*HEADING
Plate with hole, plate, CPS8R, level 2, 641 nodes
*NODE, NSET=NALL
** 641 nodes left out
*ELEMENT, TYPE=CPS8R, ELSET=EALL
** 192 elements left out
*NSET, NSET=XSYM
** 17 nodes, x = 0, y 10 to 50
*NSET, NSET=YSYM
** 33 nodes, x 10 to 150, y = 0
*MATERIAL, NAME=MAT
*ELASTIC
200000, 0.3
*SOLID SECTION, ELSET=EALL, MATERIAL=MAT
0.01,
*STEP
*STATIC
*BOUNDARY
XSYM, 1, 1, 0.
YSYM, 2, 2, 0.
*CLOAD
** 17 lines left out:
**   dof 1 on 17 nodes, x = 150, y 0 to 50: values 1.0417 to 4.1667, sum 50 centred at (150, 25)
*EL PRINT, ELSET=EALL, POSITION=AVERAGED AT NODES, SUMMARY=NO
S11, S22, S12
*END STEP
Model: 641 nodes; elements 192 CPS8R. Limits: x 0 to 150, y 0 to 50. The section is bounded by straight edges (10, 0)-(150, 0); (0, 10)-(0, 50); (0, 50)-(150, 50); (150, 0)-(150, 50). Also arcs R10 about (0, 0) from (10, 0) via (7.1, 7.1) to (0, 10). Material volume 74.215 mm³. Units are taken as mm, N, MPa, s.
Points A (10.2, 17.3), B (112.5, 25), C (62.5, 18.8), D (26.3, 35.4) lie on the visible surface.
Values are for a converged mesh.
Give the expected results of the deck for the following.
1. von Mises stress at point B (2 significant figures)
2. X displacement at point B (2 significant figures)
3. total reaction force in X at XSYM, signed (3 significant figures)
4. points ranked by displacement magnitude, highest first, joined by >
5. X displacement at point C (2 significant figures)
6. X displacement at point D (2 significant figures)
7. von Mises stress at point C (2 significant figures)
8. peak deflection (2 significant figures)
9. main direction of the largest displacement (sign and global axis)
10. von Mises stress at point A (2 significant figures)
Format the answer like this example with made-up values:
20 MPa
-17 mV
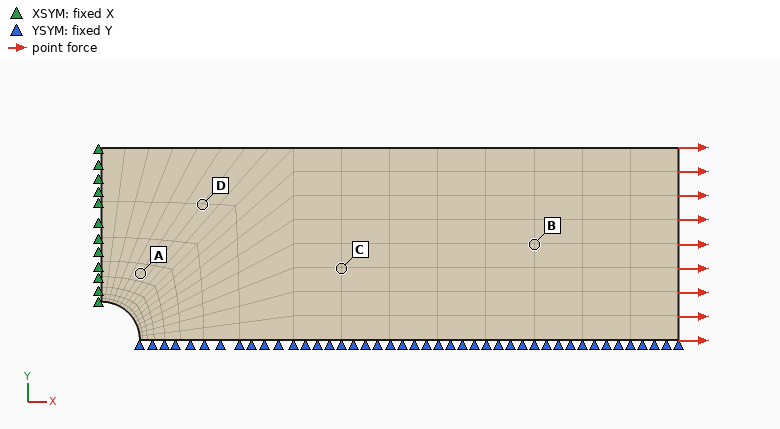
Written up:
100 MPa
0.059 mm
-50.0 N
B > C > D > A
0.034 mm
0.014 mm
97 MPa
0.079 mm
+X
130 MPa
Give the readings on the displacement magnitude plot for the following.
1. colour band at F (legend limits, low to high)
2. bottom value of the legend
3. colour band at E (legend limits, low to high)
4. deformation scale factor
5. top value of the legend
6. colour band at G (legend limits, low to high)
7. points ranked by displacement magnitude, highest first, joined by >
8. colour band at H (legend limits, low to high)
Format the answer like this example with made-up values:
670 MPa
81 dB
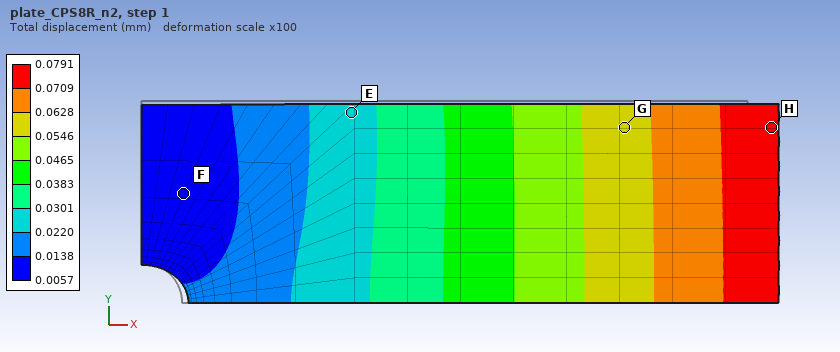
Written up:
0.0057 to 0.0138 mm
0.0057 mm
0.0220 to 0.0301 mm
100
0.0791 mm
0.0546 to 0.0628 mm
H > G > E > F
0.0709 to 0.0791 mm
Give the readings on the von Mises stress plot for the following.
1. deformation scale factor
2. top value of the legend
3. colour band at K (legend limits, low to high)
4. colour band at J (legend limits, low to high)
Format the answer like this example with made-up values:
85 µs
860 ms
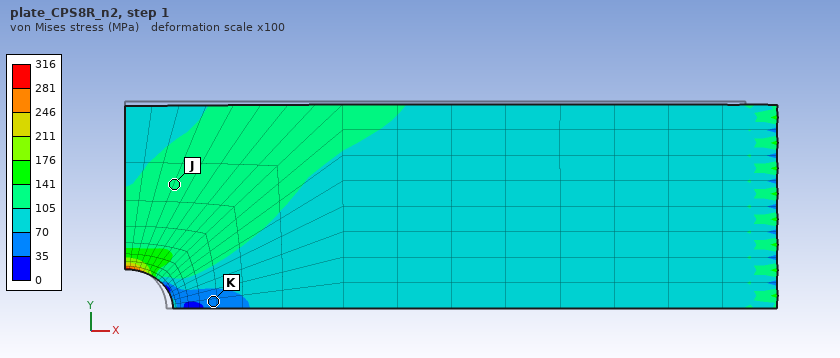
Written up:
100
316 MPa
35 to 70 MPa
105 to 141 MPa
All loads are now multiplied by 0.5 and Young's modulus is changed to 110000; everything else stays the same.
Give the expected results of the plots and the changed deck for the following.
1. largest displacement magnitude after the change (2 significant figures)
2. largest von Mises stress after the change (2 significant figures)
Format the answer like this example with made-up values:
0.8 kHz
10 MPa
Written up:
0.072 mm
160 MPa
